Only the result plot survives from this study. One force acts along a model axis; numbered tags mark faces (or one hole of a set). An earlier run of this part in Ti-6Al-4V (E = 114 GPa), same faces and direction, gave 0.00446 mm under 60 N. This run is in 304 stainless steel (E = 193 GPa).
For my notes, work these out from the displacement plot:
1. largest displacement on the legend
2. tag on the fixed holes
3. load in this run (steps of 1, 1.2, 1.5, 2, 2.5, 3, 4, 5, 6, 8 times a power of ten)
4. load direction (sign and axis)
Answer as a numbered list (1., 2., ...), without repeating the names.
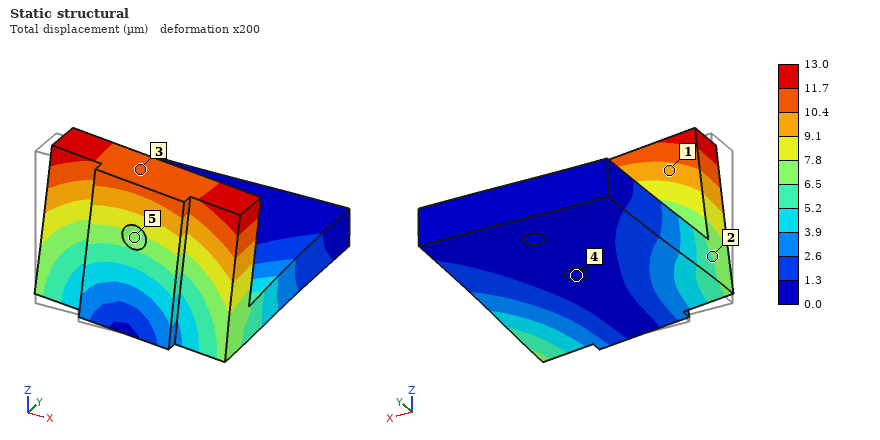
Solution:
1. 13.0 µm
2. 4
3. 300 N
4. +X
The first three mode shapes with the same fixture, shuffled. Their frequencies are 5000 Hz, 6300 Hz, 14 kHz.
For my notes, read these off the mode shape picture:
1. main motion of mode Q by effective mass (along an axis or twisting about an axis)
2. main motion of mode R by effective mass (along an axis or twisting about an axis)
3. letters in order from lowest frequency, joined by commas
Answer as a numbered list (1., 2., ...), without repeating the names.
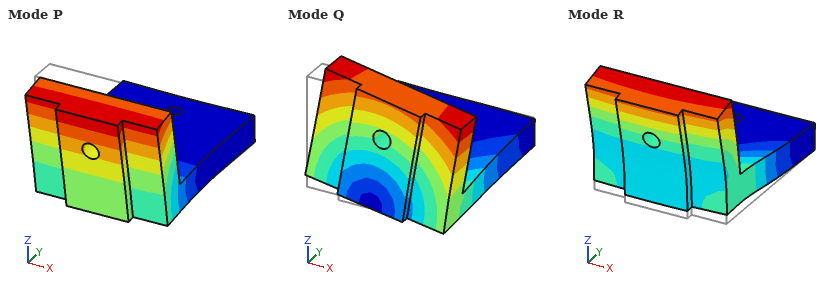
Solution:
1. along X
2. along Z
3. P, Q, R
